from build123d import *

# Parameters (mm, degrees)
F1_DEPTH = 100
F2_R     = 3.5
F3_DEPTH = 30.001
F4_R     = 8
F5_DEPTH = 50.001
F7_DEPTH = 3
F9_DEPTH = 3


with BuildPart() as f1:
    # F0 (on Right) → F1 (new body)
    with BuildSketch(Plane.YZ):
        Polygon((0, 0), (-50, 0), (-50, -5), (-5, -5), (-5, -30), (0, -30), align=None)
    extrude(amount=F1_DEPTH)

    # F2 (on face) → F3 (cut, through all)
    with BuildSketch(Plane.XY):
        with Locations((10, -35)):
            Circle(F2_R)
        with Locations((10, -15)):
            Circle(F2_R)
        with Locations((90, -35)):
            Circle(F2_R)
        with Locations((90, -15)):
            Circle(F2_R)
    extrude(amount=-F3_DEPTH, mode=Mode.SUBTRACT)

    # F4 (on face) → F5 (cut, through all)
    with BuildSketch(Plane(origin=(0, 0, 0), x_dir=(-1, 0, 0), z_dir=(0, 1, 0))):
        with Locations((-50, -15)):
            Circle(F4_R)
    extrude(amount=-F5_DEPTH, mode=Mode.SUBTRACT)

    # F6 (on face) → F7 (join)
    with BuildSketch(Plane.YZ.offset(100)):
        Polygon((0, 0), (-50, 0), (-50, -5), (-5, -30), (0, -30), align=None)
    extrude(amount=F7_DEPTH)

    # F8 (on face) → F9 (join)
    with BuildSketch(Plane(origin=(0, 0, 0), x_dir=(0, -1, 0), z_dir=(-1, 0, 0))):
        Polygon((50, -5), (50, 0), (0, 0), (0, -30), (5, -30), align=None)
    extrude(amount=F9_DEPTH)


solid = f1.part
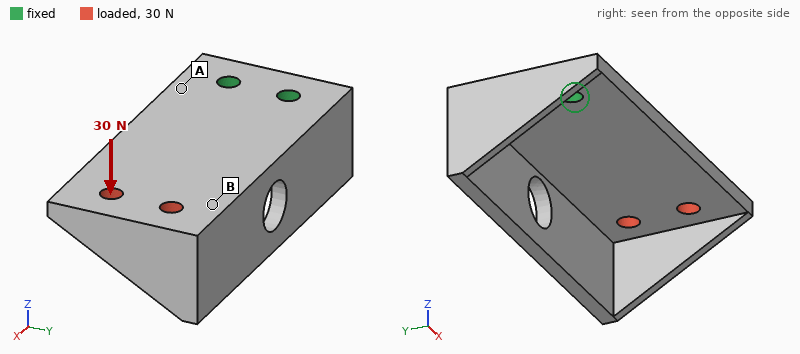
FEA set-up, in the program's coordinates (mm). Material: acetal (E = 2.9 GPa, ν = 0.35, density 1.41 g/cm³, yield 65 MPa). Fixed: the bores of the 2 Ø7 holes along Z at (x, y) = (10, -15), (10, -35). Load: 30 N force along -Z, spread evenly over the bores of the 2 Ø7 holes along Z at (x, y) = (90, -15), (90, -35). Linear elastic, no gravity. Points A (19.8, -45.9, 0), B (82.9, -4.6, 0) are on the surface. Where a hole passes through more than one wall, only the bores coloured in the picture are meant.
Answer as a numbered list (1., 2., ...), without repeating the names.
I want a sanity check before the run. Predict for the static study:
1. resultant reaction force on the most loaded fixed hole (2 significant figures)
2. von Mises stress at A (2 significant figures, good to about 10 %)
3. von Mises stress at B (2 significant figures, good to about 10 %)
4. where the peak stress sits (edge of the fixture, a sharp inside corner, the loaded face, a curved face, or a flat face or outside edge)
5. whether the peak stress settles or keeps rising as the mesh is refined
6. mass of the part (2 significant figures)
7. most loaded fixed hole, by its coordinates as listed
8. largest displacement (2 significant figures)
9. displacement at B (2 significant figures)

1. 20 N
2. 3.6 MPa
3. 1.4 MPa
4. edge of the fixture
5. keeps rising
6. 58 g
7. (10, -35)
8. 1.2 mm
9. 0.67 mm
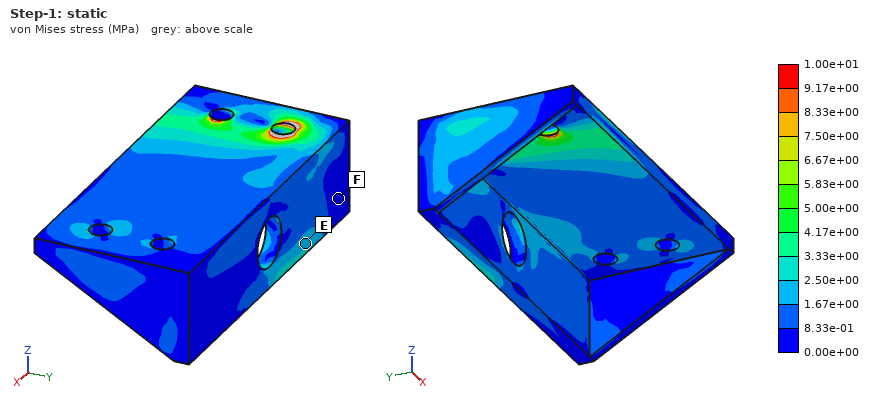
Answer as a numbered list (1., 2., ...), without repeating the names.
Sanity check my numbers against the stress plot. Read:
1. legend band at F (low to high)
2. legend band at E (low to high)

1. 0.00e+00 to 8.33e-01 MPa
2. 1.67e+00 to 2.50e+00 MPa
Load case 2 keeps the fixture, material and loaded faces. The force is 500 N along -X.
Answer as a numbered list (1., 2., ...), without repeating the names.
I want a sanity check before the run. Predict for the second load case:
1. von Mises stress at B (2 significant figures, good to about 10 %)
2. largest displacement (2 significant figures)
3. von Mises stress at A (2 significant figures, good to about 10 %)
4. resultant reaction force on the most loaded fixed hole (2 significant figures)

1. 1.3 MPa
2. 96 µm
3. 1.5 MPa
4. 250 N
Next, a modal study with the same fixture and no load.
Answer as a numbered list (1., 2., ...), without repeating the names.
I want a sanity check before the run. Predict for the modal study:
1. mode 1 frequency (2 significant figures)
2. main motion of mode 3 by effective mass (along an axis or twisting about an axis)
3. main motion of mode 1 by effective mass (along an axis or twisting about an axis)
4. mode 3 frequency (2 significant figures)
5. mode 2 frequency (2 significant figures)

1. 200 Hz
2. along Y
3. along Z
4. 770 Hz
5. 380 Hz
